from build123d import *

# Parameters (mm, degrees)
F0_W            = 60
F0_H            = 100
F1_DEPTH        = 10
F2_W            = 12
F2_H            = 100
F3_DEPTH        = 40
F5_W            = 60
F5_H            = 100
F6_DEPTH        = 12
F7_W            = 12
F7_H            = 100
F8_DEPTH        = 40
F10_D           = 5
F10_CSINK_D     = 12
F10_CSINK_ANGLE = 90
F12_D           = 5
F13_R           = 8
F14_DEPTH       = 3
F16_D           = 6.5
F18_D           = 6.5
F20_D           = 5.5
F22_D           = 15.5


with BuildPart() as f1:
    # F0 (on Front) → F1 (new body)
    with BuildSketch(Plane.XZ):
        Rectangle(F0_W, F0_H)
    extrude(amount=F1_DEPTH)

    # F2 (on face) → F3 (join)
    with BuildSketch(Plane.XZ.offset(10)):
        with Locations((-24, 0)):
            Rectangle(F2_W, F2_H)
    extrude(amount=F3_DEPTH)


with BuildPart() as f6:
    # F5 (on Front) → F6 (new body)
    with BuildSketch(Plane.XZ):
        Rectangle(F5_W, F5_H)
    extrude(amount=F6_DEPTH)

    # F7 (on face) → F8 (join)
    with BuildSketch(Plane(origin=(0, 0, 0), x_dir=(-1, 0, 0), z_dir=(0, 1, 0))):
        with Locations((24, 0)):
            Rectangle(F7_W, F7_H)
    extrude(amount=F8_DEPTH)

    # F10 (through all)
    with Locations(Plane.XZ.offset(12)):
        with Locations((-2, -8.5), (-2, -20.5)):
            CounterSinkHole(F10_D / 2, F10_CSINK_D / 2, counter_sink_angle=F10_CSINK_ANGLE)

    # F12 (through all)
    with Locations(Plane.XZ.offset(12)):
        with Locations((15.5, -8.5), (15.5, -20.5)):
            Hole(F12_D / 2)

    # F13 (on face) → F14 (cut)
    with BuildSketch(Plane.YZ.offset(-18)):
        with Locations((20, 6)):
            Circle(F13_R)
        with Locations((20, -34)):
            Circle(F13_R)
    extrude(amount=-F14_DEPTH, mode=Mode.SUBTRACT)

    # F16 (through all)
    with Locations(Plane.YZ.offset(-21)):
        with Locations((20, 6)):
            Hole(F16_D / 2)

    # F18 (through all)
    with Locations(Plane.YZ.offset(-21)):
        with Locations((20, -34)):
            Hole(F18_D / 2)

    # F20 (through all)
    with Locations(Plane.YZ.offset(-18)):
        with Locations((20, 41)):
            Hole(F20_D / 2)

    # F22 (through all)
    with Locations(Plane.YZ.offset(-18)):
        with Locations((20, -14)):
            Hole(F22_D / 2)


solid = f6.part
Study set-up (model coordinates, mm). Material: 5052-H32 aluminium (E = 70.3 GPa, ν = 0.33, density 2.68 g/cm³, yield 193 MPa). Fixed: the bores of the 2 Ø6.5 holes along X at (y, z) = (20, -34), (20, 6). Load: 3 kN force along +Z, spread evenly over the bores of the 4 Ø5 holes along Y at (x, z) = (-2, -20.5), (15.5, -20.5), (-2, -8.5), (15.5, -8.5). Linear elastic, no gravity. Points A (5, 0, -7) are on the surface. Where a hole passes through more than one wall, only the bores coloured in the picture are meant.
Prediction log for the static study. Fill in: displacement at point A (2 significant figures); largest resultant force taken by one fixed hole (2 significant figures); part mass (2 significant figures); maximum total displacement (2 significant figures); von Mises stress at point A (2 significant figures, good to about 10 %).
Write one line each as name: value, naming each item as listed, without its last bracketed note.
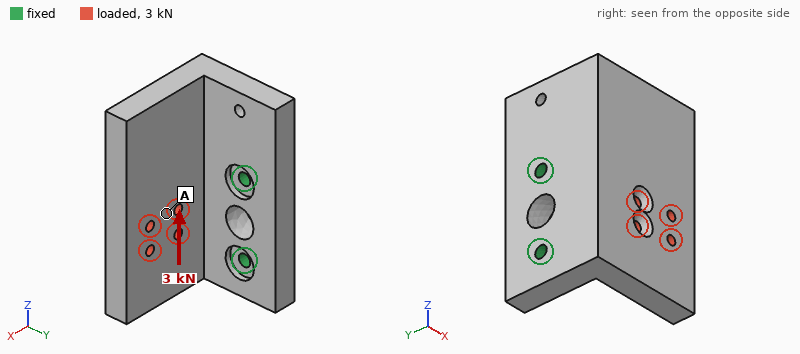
displacement at point A: 41 µm
largest resultant force taken by one fixed hole: 3.1 kN
part mass: 310 g
maximum total displacement: 97 µm
von Mises stress at point A: 11 MPa
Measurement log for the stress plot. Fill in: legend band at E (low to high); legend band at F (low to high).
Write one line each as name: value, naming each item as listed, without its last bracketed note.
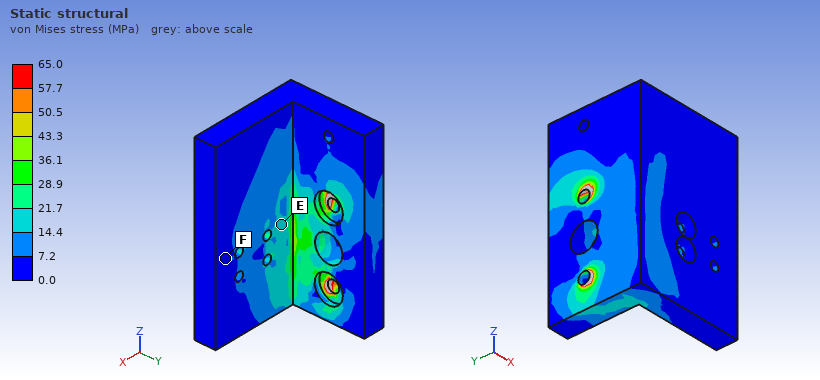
legend band at E: 14.4 to 21.7 MPa
legend band at F: 0.0 to 7.2 MPa
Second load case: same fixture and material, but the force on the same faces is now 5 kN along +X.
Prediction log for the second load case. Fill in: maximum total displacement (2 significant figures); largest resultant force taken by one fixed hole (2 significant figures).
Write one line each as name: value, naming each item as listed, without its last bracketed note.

maximum total displacement: 0.24 mm
largest resultant force taken by one fixed hole: 2.6 kN
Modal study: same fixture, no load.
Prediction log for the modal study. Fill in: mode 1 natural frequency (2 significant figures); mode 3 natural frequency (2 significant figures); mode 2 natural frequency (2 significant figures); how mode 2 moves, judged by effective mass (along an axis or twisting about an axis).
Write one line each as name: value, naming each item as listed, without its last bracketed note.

mode 1 natural frequency: 1400 Hz
mode 3 natural frequency: 3900 Hz
mode 2 natural frequency: 2400 Hz
how mode 2 moves, judged by effective mass: along Z
